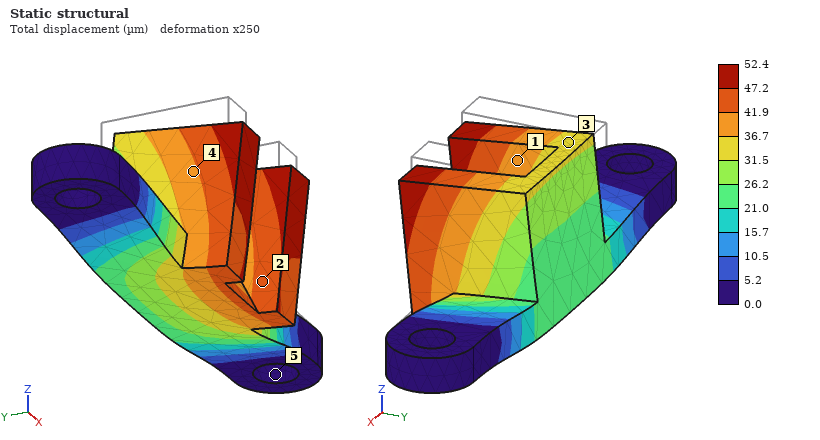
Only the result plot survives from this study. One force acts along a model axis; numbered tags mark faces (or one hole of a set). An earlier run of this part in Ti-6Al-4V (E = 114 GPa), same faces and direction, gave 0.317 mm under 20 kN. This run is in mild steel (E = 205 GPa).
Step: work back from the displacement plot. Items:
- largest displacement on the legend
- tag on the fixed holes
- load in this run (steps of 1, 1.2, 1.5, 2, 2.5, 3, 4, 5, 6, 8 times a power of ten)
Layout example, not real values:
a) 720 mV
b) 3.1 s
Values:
a) 52.4 µm
b) 5
c) 6 kN
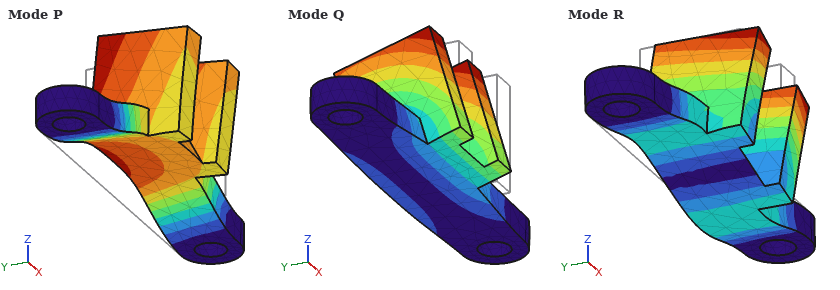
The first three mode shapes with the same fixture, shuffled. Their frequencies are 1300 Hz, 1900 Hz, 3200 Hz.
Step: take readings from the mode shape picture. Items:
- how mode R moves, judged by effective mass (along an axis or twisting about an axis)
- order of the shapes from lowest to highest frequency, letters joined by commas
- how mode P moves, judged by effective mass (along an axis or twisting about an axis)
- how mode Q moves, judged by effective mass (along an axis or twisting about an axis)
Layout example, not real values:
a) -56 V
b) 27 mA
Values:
a) along X
b) Q, P, R
c) along Z
d) along Y
